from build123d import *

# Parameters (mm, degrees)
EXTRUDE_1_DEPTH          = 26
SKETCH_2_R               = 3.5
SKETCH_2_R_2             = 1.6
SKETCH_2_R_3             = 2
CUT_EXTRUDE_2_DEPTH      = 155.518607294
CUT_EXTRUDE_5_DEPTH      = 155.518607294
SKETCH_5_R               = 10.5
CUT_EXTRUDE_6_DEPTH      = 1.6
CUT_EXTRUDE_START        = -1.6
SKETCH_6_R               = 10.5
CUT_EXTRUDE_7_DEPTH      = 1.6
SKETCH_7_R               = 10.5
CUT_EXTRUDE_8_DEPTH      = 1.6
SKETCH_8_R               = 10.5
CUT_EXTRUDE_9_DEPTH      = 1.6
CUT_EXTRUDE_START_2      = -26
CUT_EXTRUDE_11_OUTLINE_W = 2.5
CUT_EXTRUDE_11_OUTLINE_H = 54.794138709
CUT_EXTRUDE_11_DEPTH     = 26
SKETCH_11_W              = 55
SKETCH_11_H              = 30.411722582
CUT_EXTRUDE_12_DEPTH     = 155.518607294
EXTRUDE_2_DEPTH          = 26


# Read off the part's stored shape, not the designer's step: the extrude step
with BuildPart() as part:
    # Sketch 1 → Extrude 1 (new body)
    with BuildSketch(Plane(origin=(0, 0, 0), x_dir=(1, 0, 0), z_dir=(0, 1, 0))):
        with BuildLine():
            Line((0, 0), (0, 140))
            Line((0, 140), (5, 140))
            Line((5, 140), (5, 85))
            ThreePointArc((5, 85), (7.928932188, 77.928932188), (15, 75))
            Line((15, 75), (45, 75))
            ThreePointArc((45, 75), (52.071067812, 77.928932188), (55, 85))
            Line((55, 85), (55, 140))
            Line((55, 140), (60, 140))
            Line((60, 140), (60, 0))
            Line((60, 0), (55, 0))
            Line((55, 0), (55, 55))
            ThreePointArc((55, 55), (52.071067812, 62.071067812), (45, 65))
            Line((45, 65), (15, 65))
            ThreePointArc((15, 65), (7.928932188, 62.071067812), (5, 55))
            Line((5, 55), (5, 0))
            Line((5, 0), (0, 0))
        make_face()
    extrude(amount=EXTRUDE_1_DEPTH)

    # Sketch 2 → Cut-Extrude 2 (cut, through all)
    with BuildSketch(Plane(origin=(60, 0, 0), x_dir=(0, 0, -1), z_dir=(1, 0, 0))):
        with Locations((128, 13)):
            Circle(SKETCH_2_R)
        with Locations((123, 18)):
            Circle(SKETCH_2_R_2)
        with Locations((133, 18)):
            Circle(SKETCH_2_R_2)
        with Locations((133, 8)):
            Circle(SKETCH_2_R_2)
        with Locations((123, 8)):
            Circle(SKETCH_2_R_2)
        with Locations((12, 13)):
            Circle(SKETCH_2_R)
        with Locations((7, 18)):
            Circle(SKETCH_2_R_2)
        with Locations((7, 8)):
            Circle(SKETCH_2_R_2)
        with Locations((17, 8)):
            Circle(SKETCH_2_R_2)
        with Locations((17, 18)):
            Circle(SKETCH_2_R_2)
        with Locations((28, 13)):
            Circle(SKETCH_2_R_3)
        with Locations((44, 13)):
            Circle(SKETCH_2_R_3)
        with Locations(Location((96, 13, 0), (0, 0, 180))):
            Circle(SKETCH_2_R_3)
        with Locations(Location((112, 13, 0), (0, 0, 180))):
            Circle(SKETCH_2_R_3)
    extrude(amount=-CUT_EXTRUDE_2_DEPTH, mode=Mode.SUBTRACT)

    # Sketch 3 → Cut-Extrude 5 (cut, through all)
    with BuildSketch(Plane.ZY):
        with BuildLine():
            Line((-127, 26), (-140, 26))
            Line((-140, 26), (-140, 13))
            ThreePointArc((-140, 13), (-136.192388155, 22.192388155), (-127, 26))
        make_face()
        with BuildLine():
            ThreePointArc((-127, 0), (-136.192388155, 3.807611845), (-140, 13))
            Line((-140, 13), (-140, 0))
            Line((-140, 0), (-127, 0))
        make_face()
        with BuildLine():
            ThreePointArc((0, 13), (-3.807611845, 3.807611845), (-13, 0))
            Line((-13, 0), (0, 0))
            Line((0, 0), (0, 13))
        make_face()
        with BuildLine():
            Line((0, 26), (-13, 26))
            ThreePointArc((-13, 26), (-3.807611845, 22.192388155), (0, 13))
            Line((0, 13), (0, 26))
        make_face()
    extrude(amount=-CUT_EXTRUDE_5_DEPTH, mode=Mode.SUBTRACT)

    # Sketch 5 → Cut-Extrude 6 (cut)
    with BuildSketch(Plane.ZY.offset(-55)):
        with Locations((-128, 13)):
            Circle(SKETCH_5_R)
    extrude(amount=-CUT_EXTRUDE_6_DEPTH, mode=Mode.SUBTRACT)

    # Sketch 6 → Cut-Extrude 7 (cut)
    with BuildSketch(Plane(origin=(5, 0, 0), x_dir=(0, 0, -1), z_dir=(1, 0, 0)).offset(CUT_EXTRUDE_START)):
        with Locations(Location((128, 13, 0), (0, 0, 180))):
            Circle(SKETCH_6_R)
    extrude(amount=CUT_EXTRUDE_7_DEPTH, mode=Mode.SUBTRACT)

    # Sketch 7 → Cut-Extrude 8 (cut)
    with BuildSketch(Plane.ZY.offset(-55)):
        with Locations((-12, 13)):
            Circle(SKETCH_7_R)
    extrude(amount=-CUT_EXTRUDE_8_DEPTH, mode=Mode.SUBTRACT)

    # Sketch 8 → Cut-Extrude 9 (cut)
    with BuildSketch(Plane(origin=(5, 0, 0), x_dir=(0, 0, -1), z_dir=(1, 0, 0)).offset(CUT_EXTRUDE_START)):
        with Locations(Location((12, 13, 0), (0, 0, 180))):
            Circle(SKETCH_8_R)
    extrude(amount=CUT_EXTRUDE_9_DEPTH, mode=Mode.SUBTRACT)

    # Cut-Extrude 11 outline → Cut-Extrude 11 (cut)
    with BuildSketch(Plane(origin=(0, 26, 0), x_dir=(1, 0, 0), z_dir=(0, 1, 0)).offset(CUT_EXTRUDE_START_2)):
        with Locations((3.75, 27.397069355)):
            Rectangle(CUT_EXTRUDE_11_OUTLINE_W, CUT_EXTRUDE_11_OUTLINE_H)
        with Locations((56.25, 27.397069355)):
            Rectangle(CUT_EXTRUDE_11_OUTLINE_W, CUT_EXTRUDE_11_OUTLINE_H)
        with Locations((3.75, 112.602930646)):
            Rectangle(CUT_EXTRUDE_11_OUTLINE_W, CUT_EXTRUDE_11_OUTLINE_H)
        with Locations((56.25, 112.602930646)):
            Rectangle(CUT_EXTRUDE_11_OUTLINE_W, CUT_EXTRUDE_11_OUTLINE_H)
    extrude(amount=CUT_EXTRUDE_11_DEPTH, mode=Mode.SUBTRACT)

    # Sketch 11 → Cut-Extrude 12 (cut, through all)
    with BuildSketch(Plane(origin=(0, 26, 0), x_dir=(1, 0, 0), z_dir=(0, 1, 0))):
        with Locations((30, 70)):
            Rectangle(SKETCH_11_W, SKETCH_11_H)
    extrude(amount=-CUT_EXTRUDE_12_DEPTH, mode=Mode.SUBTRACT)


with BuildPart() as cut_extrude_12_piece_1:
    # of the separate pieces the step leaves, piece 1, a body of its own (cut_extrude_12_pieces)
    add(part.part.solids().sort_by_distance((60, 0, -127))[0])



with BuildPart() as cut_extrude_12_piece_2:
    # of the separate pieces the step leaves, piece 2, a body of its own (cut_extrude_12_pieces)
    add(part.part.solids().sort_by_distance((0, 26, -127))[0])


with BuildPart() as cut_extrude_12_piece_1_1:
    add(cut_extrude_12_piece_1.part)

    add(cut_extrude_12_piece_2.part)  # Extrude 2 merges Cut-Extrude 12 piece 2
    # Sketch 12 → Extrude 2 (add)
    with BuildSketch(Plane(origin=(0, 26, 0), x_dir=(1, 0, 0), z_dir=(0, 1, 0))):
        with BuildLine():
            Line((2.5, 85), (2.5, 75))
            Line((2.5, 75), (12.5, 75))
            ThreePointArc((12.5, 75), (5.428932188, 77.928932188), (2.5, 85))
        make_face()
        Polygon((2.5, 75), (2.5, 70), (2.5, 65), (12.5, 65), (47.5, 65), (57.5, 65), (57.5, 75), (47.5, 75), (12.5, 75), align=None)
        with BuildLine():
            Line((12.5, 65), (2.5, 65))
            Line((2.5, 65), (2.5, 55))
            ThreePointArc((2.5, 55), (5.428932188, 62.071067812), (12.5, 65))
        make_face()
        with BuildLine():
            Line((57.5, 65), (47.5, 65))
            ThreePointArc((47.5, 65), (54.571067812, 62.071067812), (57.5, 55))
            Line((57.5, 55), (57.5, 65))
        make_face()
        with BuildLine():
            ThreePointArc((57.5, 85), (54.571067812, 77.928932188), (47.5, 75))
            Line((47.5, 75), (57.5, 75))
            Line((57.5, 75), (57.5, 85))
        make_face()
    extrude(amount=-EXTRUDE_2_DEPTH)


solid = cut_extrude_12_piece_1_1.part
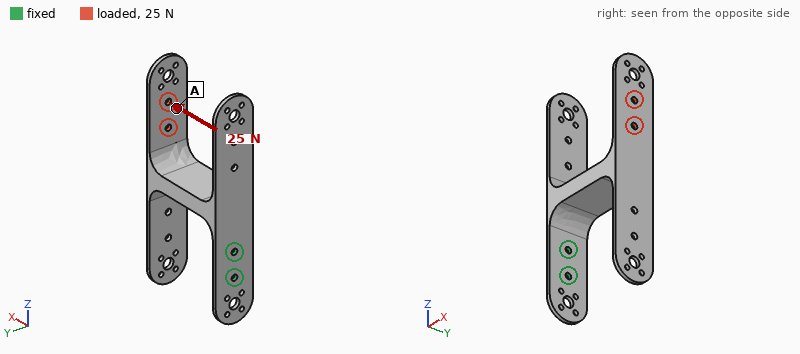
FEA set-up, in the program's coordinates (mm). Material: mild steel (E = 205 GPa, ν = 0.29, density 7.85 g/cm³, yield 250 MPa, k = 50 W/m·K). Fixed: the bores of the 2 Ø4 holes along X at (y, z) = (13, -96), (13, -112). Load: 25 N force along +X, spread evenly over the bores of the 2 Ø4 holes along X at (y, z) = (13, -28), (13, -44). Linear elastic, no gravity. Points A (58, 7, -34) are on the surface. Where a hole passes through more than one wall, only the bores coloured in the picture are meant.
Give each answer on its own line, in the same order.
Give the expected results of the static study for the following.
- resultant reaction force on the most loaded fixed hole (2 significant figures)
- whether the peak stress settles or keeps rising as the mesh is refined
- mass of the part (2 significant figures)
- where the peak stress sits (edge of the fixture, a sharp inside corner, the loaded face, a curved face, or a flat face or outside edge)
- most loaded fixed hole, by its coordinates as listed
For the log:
54 N
keeps rising
260 g
edge of the fixture
(13, -96)
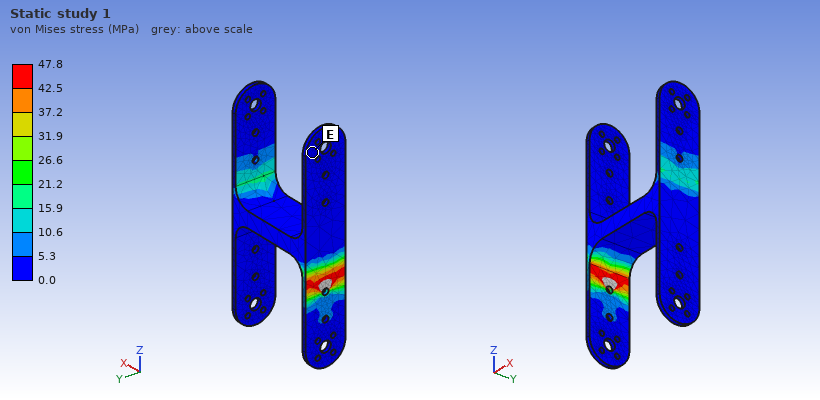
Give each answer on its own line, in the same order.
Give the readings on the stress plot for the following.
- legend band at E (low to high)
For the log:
0.0 to 5.3 MPa
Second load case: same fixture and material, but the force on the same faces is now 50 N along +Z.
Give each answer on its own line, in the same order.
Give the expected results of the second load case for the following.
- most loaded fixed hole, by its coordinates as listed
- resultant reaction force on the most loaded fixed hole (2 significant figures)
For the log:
(13, -96)
70 N
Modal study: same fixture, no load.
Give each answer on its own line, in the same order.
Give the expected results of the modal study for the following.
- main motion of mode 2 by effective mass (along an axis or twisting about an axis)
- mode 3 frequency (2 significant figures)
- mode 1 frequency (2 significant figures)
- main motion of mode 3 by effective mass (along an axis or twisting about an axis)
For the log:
along Y
640 Hz
140 Hz
along X
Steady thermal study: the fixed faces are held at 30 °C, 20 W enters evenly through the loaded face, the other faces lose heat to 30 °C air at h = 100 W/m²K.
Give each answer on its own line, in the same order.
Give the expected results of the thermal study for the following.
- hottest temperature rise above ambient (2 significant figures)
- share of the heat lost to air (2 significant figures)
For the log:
72 K
98 %
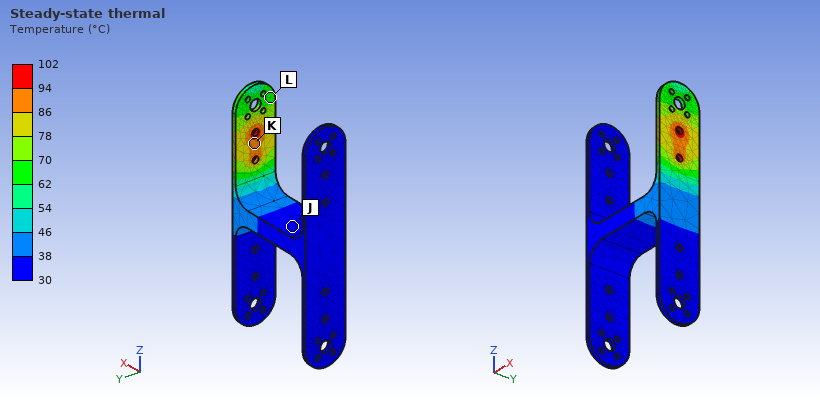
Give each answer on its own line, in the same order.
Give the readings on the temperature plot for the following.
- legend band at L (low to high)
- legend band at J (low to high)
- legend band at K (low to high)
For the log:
62 to 70 °C
30 to 38 °C
86 to 94 °C
